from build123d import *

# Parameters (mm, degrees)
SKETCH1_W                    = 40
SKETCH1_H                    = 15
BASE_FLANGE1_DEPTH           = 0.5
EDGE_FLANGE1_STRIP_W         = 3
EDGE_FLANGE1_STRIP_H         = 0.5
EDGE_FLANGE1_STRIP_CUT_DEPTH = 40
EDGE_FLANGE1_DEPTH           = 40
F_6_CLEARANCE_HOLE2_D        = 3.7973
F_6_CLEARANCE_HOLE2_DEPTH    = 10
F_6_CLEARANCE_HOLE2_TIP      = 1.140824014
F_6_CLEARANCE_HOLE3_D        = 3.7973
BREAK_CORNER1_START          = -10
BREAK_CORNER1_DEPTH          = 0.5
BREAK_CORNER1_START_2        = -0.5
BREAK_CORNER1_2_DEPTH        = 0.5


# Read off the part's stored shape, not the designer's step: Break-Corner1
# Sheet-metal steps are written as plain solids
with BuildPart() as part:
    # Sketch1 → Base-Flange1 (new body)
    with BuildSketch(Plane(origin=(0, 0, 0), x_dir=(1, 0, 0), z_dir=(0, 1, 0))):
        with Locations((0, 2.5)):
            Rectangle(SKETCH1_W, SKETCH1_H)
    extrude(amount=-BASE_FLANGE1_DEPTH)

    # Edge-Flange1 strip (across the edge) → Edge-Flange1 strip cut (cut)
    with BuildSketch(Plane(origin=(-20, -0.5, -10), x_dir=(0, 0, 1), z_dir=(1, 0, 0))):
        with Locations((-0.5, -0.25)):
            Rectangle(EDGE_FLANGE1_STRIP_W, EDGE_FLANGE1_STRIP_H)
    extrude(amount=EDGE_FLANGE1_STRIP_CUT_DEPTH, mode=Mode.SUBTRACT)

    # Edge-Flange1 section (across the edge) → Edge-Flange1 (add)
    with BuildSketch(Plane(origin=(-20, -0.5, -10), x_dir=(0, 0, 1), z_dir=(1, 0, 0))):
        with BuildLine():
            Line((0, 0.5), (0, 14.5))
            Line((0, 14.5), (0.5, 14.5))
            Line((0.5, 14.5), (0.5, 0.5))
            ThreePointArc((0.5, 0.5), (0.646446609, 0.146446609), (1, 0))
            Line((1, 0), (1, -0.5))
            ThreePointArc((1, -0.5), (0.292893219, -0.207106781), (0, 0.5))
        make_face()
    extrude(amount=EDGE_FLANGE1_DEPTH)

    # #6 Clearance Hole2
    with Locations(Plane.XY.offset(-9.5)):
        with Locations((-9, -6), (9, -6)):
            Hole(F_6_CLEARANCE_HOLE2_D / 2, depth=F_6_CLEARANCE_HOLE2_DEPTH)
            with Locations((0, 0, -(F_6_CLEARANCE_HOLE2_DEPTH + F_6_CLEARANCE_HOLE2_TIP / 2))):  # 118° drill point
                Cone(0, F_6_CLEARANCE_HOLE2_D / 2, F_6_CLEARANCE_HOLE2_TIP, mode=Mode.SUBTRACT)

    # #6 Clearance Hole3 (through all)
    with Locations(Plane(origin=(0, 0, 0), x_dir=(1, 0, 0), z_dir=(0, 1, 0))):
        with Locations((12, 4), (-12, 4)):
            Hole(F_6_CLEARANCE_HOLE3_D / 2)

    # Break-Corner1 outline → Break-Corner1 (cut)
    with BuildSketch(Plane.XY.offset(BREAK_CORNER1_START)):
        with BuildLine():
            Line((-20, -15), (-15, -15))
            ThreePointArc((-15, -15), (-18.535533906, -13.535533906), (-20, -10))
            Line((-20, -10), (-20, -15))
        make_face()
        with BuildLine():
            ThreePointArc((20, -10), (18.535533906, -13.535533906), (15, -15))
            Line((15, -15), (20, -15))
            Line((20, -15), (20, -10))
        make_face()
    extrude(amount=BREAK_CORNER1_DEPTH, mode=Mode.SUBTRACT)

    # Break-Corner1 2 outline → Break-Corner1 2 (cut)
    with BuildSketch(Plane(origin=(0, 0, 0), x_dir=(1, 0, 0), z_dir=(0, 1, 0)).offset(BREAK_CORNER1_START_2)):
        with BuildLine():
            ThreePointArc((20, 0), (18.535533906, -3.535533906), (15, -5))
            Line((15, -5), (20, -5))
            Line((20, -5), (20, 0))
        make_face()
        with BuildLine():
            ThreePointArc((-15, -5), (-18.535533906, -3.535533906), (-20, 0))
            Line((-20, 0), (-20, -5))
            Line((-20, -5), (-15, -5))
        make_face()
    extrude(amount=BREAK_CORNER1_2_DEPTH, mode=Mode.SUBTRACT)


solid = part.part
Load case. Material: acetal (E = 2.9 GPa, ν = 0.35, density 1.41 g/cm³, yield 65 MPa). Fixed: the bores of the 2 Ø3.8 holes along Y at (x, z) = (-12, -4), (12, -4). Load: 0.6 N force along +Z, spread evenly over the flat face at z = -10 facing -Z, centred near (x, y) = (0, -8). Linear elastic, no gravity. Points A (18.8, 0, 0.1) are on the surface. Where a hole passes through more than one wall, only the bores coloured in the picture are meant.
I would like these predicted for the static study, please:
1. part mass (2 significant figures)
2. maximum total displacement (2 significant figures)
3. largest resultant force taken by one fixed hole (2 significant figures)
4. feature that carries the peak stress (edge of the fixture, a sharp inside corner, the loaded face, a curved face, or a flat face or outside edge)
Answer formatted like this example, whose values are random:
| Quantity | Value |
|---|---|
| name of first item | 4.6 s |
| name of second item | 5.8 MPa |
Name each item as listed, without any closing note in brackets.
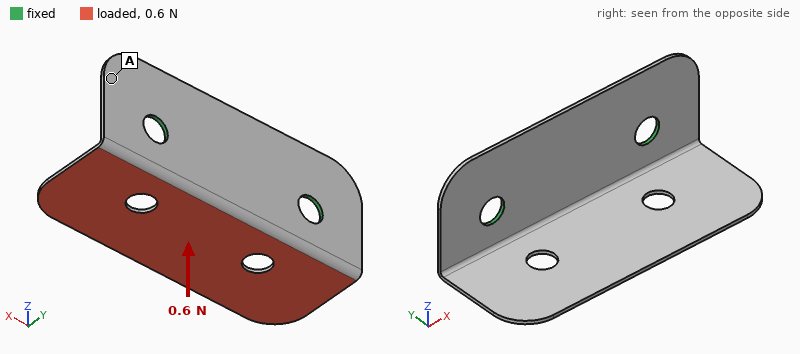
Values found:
| Quantity | Value |
|---|---|
| part mass | 0.78 g |
| maximum total displacement | 0.46 mm |
| largest resultant force taken by one fixed hole | 0.30 N |
| feature that carries the peak stress | a flat face or outside edge |
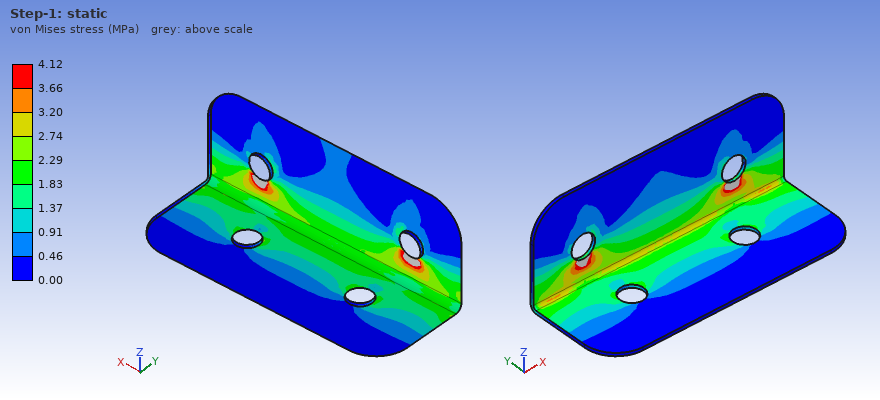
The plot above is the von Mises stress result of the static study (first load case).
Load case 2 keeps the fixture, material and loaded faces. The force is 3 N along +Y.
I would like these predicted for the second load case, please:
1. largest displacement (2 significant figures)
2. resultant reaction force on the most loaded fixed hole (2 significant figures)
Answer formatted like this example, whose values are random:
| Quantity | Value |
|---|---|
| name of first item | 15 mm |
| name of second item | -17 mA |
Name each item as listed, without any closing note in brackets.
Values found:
| Quantity | Value |
|---|---|
| largest displacement | 0.53 mm |
| resultant reaction force on the most loaded fixed hole | 1.5 N |
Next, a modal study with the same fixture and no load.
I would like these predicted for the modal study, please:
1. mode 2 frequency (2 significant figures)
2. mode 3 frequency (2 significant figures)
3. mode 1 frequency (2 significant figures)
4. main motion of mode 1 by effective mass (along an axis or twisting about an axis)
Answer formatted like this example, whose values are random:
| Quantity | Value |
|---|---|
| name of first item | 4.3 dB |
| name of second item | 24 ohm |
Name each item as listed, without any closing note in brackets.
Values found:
| Quantity | Value |
|---|---|
| mode 2 frequency | 570 Hz |
| mode 3 frequency | 1100 Hz |
| mode 1 frequency | 370 Hz |
| main motion of mode 1 by effective mass | along Z |
